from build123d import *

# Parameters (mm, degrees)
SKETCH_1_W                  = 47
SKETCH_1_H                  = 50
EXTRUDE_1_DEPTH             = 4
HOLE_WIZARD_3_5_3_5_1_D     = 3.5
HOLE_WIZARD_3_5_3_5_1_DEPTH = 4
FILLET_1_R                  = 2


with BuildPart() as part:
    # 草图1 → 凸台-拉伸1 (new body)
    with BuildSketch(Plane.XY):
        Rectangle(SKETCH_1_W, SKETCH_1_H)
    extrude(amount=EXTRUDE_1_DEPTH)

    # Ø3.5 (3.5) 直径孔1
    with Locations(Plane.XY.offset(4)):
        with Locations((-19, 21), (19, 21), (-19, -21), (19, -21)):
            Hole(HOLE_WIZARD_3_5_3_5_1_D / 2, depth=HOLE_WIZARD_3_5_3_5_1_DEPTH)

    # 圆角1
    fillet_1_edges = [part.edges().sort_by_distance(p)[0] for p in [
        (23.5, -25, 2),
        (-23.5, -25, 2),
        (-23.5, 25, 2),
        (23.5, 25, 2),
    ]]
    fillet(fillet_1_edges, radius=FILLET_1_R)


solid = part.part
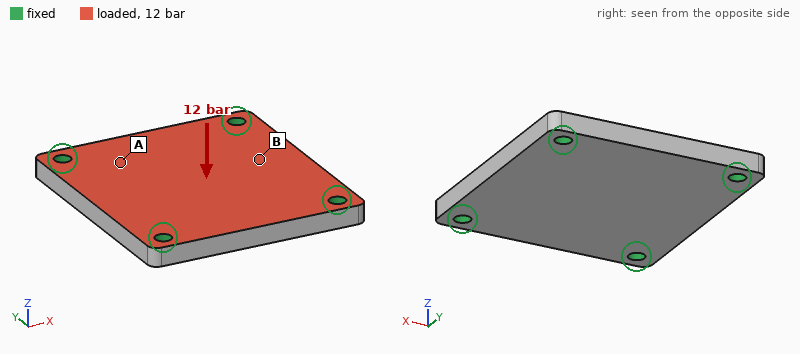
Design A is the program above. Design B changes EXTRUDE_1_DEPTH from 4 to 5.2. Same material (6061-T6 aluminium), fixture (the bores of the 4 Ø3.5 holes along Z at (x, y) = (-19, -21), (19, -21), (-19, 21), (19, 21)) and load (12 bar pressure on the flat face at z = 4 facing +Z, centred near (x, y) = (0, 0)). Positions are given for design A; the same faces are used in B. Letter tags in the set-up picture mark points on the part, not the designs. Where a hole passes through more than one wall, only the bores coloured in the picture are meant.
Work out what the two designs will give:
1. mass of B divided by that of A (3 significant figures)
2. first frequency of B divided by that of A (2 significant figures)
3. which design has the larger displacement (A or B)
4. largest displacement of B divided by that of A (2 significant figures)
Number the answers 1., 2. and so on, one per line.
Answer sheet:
1. 1.30
2. 1.2
3. A
4. 0.50
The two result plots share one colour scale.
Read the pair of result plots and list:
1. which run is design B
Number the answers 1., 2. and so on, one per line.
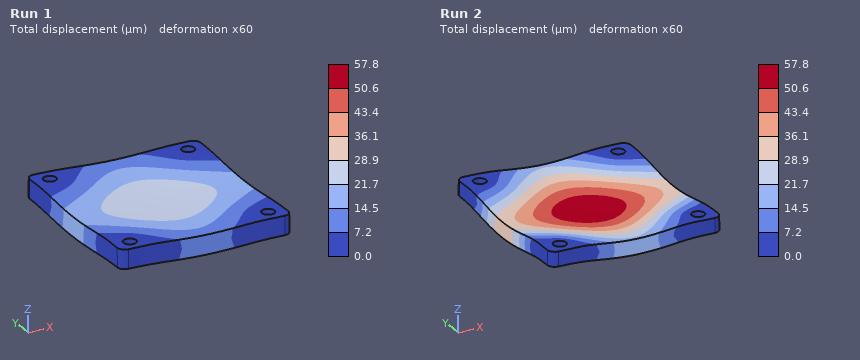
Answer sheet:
1. Run 1
